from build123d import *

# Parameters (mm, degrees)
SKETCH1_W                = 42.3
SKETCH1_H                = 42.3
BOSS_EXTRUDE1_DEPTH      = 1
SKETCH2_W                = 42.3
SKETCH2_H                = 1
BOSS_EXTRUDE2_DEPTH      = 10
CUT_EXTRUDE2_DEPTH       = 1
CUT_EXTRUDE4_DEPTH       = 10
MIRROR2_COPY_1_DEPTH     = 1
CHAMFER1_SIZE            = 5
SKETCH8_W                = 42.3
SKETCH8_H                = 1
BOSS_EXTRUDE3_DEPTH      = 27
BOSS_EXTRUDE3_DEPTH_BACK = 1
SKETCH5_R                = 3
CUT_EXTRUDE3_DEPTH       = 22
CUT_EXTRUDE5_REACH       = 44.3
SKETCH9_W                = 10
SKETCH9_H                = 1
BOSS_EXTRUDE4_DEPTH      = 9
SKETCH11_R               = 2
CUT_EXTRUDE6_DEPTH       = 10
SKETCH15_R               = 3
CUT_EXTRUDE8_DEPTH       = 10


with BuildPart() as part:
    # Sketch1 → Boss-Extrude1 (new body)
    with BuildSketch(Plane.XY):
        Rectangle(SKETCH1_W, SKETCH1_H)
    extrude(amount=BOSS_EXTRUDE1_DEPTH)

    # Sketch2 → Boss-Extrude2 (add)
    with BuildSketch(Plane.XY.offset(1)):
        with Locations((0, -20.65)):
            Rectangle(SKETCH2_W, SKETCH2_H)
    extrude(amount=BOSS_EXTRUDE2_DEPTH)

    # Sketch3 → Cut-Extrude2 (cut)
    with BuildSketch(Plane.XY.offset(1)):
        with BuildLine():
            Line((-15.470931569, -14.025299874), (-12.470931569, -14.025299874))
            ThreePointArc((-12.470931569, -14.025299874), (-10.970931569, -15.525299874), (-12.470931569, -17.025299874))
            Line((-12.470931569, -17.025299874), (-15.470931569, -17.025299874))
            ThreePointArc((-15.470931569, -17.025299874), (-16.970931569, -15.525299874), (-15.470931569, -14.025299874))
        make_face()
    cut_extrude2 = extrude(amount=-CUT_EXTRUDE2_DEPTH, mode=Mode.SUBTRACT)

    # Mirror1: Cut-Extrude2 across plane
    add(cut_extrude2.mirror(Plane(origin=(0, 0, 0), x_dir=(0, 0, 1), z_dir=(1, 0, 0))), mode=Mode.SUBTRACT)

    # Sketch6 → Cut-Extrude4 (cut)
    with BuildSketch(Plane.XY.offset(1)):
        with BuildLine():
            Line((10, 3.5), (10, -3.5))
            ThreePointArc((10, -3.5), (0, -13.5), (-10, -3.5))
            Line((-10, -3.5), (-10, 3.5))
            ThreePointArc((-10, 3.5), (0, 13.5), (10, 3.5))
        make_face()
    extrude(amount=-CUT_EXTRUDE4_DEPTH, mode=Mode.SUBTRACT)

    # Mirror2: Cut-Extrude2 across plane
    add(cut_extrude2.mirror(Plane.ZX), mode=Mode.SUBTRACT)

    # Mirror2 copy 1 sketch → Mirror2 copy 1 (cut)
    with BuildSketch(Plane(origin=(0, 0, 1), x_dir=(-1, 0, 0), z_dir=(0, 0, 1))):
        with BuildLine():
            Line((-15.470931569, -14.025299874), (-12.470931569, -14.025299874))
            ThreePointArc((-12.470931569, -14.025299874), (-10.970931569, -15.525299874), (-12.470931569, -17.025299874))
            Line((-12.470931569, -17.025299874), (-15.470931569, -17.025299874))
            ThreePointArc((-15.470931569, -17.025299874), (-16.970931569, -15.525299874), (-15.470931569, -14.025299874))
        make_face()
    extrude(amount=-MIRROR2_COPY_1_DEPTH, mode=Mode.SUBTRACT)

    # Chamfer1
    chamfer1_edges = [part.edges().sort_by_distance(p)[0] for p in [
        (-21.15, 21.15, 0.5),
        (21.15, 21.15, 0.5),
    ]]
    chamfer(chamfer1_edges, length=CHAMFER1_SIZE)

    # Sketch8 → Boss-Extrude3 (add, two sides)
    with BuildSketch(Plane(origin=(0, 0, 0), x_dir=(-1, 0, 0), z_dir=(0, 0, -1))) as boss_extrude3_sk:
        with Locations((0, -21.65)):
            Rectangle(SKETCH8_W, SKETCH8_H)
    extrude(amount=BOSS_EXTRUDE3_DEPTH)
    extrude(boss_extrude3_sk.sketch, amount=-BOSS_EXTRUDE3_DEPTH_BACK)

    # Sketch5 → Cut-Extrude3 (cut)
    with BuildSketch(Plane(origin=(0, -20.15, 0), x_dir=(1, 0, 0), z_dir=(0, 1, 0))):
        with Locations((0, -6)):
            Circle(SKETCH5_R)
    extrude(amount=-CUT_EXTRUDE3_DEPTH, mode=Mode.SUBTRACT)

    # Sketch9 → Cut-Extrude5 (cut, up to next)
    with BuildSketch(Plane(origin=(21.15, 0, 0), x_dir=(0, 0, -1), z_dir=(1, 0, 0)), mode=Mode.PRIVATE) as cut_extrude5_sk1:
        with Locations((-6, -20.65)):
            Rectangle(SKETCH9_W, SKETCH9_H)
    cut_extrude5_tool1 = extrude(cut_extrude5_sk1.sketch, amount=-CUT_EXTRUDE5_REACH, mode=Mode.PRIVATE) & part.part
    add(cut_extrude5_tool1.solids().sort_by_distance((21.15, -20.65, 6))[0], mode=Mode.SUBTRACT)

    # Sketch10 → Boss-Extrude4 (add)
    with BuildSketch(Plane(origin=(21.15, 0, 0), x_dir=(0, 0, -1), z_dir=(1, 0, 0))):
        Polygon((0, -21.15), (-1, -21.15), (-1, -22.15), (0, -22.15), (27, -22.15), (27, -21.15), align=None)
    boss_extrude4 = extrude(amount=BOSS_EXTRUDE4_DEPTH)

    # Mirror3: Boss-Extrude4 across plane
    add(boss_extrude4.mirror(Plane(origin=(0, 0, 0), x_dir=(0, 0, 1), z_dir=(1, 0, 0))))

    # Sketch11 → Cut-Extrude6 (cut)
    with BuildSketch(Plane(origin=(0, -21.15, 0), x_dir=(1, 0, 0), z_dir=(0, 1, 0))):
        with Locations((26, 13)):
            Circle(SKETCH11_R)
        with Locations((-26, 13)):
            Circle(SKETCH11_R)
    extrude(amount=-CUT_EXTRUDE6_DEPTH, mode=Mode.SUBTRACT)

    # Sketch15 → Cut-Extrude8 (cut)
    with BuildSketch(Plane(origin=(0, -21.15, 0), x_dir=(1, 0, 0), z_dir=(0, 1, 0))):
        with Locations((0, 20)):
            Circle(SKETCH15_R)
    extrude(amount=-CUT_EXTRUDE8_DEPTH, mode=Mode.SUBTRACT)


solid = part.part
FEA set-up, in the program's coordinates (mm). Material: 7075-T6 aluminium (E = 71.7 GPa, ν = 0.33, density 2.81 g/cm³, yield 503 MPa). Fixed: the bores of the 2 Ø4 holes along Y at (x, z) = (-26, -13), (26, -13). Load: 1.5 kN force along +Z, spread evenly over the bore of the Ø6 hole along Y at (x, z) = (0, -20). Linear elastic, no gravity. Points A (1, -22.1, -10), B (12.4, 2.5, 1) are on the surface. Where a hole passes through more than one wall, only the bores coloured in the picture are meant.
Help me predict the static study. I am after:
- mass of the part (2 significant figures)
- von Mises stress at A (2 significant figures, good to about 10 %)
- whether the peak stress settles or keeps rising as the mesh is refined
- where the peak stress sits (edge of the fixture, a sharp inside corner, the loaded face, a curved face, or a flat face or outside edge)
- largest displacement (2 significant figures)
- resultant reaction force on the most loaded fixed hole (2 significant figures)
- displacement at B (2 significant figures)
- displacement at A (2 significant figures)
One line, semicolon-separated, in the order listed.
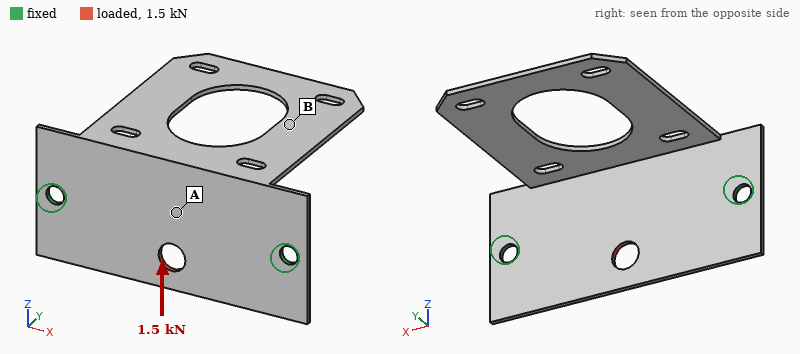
8.1 g; 53 MPa; keeps rising; edge of the fixture; 75 µm; 750 N; 53 µm; 48 µm
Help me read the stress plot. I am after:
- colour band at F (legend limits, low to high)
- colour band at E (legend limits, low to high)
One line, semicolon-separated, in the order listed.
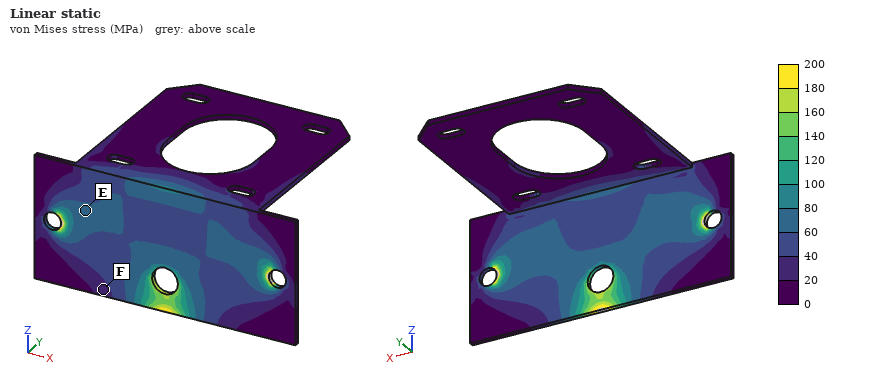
20 to 40 MPa; 60 to 80 MPa
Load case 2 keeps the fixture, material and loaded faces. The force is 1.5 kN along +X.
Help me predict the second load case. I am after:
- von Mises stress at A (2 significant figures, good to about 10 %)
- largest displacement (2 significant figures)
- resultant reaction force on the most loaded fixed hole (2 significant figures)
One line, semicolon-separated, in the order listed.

18 MPa; 24 µm; 770 N
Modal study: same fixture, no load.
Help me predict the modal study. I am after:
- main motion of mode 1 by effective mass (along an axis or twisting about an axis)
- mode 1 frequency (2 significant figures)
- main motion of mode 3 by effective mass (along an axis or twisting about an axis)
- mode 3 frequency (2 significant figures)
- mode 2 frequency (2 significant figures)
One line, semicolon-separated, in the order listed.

along Z; 320 Hz; along X; 1300 Hz; 880 Hz
